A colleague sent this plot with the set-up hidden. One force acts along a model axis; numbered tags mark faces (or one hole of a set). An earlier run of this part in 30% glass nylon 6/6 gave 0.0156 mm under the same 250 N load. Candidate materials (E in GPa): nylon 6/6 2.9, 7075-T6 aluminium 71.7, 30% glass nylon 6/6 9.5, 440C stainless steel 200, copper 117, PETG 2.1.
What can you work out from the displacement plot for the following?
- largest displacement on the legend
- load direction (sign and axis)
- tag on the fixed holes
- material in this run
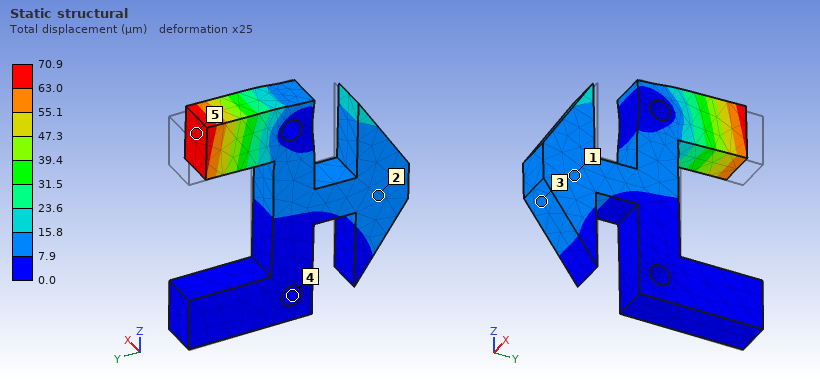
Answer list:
70.9 µm
-Y
4
PETG
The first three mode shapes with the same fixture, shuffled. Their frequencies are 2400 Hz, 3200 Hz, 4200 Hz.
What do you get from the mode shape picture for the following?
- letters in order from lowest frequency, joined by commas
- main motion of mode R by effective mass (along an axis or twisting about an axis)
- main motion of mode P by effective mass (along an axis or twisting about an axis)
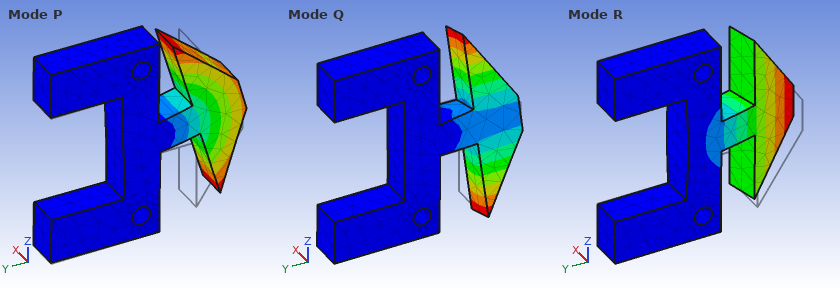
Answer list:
R, P, Q
along X
along Z
